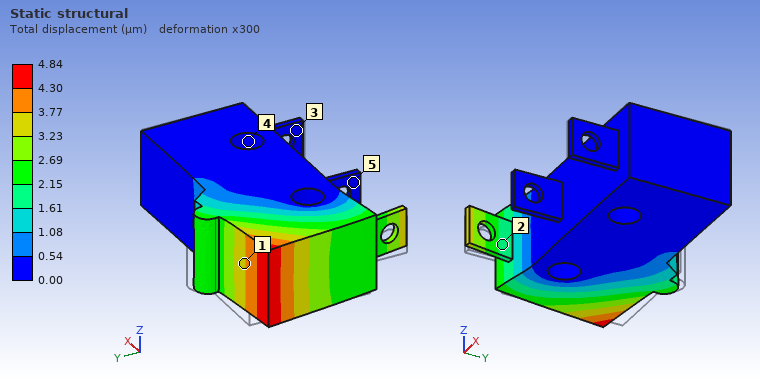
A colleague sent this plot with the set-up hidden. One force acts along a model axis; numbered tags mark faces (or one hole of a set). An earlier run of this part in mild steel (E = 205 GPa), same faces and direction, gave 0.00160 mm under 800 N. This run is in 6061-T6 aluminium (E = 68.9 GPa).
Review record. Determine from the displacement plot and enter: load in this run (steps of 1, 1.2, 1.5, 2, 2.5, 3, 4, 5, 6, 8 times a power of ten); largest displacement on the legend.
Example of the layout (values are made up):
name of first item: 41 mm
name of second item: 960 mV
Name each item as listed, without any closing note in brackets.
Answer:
load in this run: 800 N
largest displacement on the legend: 4.84 µm
